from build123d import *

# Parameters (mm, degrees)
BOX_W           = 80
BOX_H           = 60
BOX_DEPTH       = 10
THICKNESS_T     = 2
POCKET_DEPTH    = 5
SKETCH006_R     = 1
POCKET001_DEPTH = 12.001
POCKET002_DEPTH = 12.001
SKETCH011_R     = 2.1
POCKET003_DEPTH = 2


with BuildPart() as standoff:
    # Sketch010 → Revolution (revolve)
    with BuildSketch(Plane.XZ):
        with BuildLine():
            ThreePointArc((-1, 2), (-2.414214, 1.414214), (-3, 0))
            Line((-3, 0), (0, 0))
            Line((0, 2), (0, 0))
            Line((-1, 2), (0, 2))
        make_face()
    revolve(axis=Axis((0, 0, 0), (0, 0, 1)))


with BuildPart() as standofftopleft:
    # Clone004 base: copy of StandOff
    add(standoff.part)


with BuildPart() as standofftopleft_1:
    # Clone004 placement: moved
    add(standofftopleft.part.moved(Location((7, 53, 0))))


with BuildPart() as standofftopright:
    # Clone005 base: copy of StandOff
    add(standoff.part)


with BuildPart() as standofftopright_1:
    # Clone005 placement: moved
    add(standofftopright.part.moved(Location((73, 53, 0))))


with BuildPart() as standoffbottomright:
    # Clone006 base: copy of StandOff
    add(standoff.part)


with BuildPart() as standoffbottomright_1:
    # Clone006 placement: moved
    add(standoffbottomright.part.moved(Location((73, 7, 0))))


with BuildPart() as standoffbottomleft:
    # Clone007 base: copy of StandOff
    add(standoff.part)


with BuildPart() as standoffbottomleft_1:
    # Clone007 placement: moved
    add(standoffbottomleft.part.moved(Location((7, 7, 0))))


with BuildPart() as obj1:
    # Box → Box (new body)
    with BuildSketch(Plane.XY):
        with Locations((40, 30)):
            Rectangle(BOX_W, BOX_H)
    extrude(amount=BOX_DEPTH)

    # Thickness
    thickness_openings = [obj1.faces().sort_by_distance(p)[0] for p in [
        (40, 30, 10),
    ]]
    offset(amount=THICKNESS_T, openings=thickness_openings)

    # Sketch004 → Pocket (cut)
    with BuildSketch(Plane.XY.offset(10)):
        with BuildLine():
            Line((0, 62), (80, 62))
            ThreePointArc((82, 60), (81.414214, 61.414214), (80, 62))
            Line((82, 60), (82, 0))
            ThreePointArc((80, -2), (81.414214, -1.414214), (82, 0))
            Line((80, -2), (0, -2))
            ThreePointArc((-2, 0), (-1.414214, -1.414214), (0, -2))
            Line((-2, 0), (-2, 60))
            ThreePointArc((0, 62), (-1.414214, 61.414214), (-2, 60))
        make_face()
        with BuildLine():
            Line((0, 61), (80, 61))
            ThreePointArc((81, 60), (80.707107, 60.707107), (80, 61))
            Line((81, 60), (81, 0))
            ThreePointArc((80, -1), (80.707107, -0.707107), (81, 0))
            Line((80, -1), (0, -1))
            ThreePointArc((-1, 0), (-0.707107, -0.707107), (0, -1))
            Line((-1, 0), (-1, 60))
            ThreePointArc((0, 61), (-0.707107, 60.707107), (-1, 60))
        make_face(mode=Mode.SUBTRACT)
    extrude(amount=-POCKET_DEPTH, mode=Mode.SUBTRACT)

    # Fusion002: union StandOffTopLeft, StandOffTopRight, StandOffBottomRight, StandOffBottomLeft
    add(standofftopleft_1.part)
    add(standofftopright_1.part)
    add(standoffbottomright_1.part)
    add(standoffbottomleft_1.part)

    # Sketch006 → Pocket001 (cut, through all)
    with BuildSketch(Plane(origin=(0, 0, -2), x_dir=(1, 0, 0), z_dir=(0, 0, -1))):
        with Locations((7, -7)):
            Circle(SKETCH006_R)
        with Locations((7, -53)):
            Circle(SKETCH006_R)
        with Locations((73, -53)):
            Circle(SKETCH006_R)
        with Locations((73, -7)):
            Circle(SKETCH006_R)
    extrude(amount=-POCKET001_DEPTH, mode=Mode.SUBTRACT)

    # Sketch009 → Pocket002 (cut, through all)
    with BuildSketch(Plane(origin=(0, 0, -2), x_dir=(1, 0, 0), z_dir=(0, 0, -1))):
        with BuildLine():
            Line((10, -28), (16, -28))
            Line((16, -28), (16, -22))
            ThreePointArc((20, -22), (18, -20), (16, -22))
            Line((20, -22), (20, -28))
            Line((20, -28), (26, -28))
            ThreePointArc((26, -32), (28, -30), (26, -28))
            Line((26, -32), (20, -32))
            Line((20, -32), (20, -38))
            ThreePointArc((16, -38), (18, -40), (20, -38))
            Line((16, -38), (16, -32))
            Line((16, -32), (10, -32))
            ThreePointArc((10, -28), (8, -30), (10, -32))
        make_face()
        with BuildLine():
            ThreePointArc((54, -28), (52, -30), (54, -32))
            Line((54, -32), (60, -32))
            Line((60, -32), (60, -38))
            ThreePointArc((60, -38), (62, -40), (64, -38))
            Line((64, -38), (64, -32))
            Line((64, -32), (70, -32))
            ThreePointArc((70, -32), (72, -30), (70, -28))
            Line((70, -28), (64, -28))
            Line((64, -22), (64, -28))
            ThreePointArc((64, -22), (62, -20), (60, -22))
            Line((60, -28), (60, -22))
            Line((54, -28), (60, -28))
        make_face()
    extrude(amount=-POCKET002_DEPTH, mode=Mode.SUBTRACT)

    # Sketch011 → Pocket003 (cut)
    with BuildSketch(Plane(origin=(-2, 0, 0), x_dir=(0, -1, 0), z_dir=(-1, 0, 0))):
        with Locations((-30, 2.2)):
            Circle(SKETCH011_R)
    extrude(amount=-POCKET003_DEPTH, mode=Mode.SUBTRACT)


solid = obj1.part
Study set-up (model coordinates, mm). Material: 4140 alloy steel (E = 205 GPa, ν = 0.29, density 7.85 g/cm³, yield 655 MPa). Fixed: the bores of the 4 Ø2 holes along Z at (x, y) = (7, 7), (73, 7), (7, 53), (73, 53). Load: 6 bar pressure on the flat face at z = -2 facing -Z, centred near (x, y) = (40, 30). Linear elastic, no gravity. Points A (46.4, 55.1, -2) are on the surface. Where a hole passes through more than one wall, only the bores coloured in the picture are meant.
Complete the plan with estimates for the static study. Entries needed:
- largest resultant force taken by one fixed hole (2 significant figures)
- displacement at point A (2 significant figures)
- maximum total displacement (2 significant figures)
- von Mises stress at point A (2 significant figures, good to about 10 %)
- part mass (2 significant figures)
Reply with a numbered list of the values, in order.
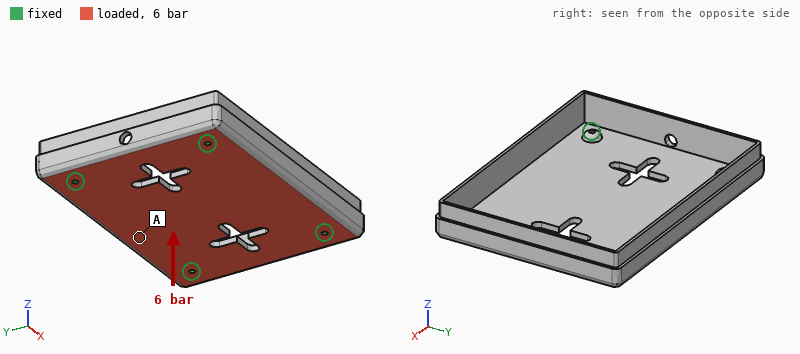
1. 700 N
2. 0.070 mm
3. 0.22 mm
4. 58 MPa
5. 110 g
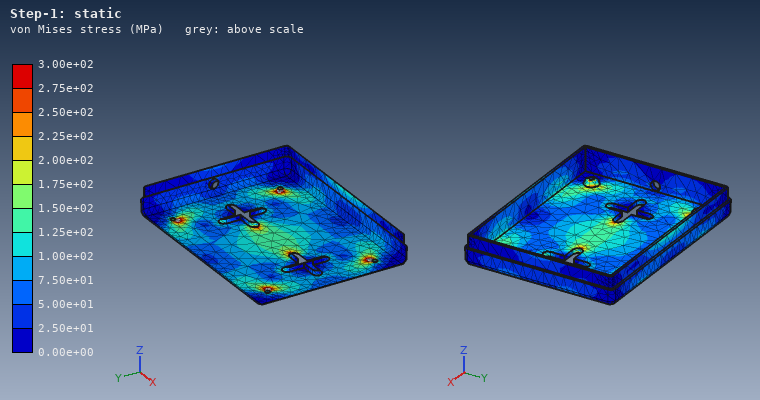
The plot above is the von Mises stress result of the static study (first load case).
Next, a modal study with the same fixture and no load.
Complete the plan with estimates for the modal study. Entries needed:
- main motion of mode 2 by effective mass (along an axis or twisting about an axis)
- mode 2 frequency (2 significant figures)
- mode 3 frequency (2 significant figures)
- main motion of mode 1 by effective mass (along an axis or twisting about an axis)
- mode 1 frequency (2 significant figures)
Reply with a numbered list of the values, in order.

1. twisting about X
2. 5000 Hz
3. 5300 Hz
4. along Z
5. 2600 Hz
